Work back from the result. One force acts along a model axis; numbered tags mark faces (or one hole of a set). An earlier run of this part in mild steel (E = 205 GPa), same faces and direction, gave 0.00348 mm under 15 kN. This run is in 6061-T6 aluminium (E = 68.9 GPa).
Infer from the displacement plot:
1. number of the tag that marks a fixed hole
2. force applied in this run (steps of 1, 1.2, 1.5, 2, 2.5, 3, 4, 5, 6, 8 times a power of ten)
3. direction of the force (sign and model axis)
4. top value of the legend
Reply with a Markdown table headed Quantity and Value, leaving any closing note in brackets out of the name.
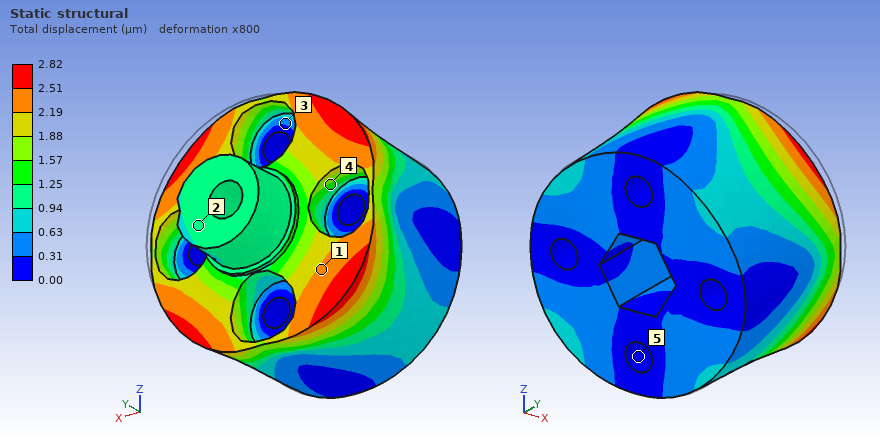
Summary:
| Quantity | Value |
|---|---|
| number of the tag that marks a fixed hole | 5 |
| force applied in this run | 4 kN |
| direction of the force | -Y |
| top value of the legend | 2.82 µm |
